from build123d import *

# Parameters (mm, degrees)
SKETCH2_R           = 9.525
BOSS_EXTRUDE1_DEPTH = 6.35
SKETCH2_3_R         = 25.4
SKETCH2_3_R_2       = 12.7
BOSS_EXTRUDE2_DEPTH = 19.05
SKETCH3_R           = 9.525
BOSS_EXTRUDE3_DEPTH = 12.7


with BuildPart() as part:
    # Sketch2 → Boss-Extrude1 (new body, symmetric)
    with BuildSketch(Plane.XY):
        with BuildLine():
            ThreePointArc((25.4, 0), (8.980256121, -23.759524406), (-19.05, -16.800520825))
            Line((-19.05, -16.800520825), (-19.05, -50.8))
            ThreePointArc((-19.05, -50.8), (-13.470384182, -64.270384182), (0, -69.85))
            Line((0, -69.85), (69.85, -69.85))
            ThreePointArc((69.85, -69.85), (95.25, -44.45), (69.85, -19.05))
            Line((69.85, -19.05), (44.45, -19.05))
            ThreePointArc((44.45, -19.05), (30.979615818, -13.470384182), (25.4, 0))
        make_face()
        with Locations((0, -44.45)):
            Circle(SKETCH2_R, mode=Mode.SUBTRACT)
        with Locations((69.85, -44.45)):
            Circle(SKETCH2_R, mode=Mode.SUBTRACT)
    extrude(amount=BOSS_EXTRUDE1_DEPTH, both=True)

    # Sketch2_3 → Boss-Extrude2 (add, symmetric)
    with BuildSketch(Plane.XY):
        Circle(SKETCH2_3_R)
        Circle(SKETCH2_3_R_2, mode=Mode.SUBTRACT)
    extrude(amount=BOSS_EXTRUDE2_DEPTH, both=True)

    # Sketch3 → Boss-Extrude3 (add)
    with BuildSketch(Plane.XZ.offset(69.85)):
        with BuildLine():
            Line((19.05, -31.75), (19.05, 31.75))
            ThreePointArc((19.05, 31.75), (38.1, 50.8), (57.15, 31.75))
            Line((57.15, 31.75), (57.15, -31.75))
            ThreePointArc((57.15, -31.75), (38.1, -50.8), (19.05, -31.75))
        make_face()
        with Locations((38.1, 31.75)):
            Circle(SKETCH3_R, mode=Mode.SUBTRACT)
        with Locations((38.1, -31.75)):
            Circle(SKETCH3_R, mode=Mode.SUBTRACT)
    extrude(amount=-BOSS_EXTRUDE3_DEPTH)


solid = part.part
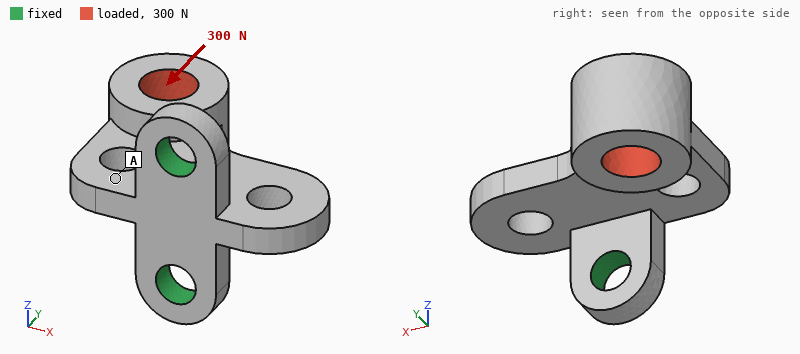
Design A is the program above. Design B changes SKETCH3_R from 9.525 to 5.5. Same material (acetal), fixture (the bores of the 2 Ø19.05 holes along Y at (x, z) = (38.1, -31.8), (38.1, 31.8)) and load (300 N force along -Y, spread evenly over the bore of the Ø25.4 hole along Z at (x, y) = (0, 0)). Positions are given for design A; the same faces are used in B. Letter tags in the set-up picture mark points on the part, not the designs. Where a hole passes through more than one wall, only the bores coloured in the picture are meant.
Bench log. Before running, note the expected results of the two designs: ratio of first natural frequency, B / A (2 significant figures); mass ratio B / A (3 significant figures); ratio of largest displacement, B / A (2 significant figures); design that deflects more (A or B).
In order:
0.98
1.03
1.3
B
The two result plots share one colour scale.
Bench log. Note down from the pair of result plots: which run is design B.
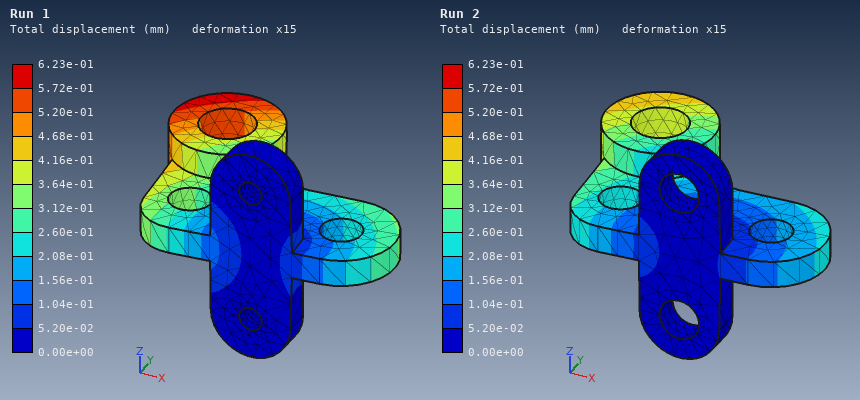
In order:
Run 1
